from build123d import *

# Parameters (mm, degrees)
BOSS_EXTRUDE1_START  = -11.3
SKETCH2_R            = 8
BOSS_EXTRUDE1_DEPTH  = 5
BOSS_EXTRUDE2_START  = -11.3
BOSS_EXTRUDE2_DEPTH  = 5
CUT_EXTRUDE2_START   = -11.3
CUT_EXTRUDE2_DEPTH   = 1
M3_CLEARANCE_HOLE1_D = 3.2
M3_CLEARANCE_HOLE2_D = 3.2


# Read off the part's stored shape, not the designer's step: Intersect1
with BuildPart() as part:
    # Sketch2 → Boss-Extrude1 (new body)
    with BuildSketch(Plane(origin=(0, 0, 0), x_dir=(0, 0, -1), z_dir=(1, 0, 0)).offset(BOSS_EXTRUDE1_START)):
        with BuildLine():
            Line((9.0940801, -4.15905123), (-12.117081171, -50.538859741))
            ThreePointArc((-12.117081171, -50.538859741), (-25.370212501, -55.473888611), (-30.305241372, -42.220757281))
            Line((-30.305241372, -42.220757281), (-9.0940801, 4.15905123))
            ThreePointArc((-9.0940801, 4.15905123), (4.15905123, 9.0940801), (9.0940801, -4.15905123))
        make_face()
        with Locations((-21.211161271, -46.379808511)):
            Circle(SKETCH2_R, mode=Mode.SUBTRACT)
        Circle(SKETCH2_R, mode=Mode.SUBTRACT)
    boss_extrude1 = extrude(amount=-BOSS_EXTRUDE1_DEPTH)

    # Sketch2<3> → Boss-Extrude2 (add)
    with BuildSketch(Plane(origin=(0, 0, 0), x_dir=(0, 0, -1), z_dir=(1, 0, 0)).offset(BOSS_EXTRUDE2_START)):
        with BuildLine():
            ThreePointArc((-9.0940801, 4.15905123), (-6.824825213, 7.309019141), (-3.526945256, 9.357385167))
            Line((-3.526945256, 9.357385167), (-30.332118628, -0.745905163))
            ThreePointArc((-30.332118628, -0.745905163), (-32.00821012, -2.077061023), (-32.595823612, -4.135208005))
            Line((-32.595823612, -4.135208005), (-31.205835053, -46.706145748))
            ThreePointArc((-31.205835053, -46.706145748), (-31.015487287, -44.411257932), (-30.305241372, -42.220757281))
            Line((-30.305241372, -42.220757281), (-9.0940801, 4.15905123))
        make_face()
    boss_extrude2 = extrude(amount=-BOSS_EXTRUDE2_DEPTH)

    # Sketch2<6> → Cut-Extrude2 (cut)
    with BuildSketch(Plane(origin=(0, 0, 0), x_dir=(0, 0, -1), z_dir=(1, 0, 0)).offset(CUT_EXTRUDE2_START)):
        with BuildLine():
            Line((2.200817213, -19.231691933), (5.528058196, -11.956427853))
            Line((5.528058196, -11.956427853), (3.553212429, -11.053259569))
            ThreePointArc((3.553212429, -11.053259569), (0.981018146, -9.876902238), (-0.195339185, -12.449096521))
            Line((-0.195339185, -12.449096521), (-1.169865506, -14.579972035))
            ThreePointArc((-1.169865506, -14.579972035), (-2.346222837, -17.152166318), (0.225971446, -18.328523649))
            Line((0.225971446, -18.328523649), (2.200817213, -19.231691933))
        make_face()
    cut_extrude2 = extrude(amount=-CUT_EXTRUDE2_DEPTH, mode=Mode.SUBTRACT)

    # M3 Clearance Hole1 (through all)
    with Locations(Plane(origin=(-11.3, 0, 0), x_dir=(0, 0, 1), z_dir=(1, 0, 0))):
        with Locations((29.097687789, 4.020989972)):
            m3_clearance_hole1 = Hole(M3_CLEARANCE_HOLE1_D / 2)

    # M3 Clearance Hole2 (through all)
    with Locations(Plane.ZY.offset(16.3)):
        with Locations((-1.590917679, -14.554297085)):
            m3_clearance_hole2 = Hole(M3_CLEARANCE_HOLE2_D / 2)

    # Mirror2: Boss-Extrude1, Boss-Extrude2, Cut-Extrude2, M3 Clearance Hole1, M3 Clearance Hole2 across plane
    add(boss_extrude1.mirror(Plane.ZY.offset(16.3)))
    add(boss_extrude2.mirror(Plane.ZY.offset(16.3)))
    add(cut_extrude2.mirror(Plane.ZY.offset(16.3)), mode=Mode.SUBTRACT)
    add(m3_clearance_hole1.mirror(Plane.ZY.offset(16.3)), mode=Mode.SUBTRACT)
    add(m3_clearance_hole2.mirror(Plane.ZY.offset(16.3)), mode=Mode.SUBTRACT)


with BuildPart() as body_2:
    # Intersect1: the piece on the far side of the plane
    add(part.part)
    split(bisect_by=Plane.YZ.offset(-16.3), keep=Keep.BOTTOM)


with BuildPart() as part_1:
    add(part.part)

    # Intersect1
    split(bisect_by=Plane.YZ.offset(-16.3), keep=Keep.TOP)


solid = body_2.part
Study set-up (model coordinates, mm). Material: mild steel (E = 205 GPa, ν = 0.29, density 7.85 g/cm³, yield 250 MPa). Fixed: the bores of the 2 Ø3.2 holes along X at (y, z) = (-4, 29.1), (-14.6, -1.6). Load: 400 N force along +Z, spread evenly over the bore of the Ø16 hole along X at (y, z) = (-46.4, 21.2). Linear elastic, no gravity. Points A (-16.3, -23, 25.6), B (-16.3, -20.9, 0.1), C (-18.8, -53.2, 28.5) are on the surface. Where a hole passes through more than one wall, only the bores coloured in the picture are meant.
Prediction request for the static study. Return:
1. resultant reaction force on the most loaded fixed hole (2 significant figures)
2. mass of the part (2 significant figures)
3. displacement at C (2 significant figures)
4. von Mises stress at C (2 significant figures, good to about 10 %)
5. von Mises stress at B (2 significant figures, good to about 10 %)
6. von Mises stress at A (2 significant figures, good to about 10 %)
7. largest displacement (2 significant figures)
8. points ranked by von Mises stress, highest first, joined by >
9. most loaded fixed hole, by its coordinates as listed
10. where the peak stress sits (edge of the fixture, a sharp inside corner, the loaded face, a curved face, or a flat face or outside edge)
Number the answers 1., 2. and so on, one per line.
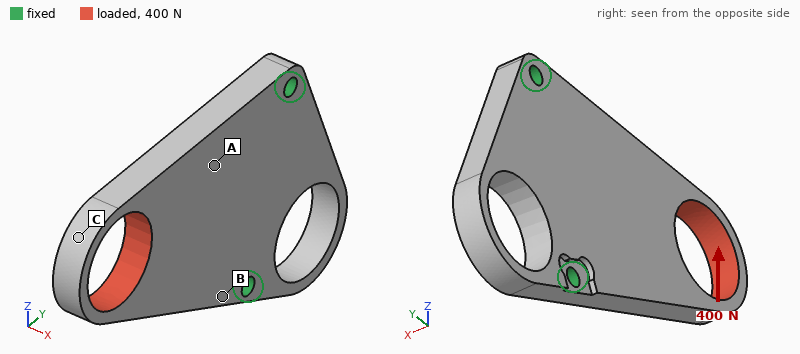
1. 550 N
2. 57 g
3. 16 µm
4. 42 MPa
5. 16 MPa
6. 6.4 MPa
7. 16 µm
8. C > B > A
9. (-14.6, -1.6)
10. the loaded face
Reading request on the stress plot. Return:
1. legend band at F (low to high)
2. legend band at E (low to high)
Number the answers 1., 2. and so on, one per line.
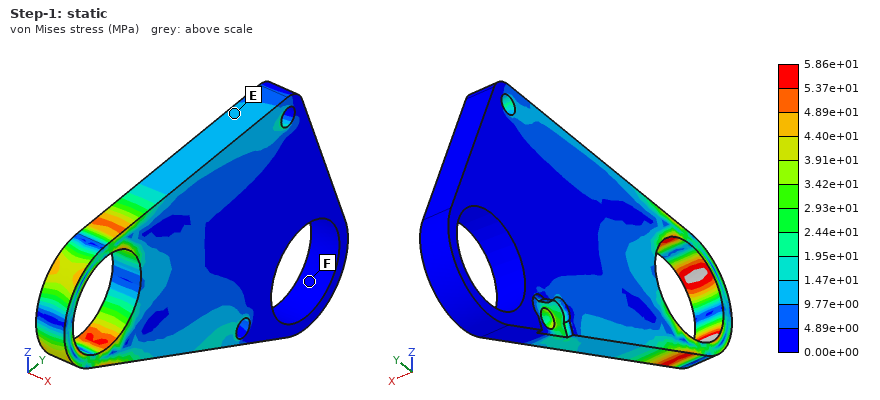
1. 0.00e+00 to 4.89e+00 MPa
2. 9.77e+00 to 1.47e+01 MPa
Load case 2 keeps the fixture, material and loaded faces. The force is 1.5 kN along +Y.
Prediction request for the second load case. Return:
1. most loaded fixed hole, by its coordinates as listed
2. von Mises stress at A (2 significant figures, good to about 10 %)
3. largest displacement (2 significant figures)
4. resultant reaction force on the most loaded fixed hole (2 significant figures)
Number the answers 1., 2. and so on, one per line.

1. (-4, 29.1)
2. 14 MPa
3. 16 µm
4. 1.1 kN
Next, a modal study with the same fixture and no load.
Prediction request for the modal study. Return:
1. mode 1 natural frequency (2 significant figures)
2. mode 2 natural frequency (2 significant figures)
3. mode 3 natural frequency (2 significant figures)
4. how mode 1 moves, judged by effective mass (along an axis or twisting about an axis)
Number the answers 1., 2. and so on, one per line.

1. 2700 Hz
2. 8600 Hz
3. 9500 Hz
4. along X
